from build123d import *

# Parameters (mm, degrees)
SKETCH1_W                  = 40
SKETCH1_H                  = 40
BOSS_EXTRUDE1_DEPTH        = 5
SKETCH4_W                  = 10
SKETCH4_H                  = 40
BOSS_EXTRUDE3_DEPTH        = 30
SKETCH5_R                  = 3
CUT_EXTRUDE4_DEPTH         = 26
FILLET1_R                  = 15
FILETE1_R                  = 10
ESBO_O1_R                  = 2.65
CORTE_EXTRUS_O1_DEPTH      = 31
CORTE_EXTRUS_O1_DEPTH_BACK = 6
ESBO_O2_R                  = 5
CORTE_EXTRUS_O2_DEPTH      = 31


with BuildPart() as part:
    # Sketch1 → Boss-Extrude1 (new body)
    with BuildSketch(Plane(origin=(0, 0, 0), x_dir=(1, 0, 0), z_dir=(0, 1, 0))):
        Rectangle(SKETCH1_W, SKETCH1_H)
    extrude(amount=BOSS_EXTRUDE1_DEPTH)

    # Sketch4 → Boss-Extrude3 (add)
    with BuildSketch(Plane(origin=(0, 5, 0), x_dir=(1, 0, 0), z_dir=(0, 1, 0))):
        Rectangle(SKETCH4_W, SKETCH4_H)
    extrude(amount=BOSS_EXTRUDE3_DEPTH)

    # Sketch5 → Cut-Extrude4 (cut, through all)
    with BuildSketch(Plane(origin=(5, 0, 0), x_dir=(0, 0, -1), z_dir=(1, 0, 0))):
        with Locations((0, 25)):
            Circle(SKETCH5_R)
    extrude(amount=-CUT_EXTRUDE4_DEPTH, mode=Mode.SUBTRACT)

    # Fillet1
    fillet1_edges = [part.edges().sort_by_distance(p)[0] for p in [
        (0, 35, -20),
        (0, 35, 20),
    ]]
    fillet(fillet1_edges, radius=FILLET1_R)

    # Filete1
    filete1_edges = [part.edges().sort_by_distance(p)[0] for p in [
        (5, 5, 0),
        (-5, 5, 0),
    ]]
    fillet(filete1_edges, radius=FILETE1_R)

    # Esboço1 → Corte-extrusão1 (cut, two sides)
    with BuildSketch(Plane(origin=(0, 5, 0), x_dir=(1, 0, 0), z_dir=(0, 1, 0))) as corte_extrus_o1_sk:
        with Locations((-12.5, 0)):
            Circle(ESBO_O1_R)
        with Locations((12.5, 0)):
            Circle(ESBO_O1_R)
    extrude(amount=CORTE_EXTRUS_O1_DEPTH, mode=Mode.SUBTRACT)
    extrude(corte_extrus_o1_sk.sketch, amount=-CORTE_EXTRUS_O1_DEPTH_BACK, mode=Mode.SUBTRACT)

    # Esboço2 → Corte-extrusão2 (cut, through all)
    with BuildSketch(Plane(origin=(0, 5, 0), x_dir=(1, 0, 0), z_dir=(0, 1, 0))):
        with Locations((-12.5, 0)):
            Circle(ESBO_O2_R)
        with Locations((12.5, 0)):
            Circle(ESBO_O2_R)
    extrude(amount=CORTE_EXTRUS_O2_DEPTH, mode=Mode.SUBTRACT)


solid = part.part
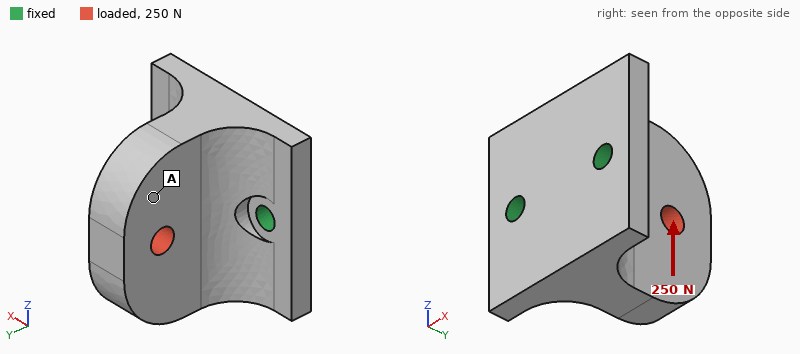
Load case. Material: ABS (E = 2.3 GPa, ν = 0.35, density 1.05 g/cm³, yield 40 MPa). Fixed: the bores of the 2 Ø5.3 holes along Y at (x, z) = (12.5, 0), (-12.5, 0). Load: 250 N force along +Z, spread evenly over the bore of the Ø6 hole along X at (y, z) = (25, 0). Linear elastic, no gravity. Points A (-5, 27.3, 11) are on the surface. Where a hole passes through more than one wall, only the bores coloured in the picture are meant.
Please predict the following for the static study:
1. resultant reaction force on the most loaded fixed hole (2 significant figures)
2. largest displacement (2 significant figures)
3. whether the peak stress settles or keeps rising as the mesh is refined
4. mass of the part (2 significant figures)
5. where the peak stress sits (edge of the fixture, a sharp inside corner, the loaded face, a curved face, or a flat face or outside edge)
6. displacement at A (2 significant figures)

130 N
0.49 mm
keeps rising
21 g
edge of the fixture
0.40 mm
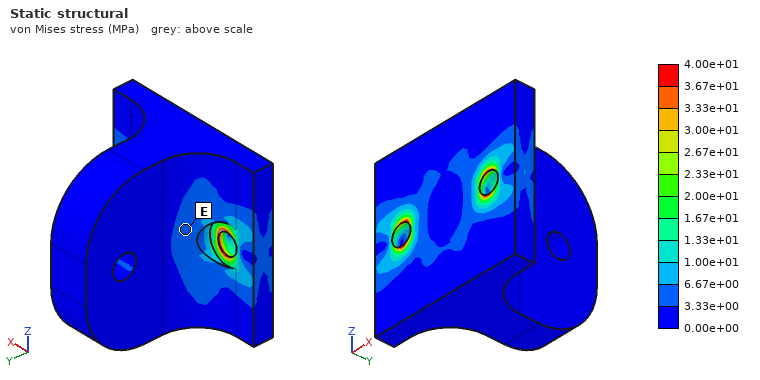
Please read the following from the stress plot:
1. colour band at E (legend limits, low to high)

3.33e+00 to 6.67e+00 MPa
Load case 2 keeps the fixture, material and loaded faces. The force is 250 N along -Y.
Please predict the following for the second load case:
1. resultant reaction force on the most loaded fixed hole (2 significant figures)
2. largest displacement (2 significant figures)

130 N
30 µm
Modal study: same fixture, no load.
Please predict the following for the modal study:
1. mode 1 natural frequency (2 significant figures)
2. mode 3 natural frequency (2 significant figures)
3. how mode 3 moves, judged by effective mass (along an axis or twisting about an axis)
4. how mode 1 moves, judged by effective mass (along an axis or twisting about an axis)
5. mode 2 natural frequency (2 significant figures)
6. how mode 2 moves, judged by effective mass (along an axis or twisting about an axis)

1300 Hz
4300 Hz
along Y
along Z
2600 Hz
along X
